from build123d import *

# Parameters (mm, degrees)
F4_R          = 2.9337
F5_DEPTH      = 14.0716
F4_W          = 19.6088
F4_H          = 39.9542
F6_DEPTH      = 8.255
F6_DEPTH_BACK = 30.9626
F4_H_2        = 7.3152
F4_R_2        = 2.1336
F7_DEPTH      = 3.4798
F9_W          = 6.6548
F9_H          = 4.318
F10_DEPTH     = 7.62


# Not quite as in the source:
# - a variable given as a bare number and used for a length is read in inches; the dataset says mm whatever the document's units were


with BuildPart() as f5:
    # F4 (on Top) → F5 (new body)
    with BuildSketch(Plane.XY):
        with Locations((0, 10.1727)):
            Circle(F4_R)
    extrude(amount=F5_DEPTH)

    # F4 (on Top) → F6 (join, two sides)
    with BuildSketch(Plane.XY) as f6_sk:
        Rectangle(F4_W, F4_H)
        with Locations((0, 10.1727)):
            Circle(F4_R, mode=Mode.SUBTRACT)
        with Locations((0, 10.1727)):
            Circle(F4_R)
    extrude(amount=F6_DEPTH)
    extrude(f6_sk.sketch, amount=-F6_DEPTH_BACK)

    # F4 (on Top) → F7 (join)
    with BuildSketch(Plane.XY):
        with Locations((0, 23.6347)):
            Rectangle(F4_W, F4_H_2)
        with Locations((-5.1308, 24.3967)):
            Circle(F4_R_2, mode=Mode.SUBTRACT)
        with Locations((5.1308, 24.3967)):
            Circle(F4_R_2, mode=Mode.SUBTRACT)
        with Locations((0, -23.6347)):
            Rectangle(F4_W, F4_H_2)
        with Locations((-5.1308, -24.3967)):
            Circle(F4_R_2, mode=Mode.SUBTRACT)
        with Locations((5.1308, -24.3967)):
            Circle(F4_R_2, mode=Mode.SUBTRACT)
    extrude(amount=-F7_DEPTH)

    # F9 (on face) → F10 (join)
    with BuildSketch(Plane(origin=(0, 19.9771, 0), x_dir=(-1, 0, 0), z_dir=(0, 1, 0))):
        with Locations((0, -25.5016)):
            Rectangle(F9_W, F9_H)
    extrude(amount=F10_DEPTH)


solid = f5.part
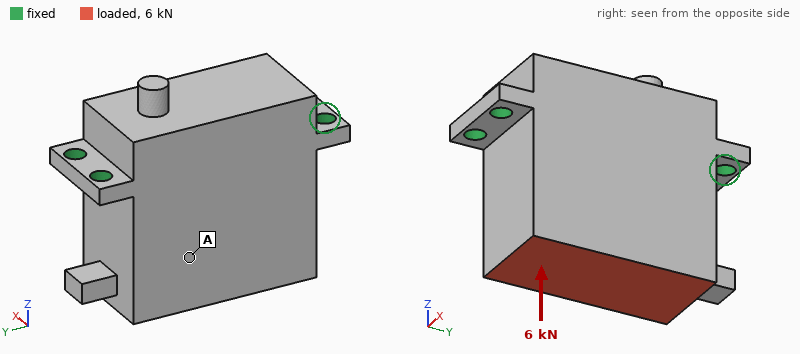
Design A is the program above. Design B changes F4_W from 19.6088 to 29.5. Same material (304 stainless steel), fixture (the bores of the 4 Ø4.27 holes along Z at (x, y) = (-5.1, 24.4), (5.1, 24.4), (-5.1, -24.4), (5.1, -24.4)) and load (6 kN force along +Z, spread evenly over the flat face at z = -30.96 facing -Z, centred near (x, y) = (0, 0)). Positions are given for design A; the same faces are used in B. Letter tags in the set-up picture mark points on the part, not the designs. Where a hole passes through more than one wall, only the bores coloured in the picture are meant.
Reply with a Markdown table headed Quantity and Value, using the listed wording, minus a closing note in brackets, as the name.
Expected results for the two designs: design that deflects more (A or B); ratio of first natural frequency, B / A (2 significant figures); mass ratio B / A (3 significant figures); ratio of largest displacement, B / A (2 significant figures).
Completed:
| Quantity | Value |
|---|---|
| design that deflects more | A |
| ratio of first natural frequency, B / A | 0.89 |
| mass ratio B / A | 1.50 |
| ratio of largest displacement, B / A | 0.85 |
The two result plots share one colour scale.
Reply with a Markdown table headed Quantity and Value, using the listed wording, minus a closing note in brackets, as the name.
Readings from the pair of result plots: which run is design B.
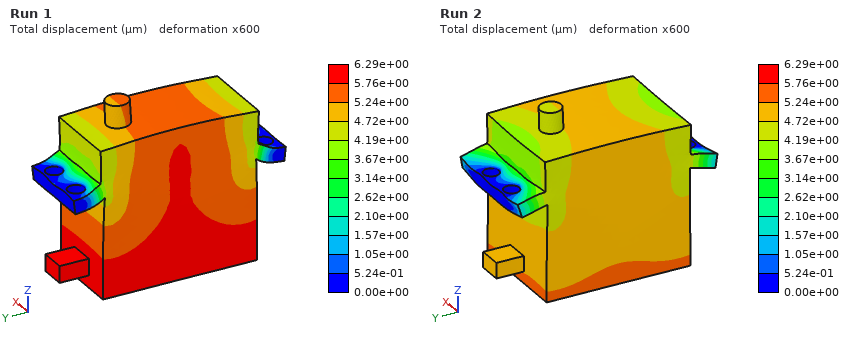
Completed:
| Quantity | Value |
|---|---|
| which run is design B | Run 2 |
